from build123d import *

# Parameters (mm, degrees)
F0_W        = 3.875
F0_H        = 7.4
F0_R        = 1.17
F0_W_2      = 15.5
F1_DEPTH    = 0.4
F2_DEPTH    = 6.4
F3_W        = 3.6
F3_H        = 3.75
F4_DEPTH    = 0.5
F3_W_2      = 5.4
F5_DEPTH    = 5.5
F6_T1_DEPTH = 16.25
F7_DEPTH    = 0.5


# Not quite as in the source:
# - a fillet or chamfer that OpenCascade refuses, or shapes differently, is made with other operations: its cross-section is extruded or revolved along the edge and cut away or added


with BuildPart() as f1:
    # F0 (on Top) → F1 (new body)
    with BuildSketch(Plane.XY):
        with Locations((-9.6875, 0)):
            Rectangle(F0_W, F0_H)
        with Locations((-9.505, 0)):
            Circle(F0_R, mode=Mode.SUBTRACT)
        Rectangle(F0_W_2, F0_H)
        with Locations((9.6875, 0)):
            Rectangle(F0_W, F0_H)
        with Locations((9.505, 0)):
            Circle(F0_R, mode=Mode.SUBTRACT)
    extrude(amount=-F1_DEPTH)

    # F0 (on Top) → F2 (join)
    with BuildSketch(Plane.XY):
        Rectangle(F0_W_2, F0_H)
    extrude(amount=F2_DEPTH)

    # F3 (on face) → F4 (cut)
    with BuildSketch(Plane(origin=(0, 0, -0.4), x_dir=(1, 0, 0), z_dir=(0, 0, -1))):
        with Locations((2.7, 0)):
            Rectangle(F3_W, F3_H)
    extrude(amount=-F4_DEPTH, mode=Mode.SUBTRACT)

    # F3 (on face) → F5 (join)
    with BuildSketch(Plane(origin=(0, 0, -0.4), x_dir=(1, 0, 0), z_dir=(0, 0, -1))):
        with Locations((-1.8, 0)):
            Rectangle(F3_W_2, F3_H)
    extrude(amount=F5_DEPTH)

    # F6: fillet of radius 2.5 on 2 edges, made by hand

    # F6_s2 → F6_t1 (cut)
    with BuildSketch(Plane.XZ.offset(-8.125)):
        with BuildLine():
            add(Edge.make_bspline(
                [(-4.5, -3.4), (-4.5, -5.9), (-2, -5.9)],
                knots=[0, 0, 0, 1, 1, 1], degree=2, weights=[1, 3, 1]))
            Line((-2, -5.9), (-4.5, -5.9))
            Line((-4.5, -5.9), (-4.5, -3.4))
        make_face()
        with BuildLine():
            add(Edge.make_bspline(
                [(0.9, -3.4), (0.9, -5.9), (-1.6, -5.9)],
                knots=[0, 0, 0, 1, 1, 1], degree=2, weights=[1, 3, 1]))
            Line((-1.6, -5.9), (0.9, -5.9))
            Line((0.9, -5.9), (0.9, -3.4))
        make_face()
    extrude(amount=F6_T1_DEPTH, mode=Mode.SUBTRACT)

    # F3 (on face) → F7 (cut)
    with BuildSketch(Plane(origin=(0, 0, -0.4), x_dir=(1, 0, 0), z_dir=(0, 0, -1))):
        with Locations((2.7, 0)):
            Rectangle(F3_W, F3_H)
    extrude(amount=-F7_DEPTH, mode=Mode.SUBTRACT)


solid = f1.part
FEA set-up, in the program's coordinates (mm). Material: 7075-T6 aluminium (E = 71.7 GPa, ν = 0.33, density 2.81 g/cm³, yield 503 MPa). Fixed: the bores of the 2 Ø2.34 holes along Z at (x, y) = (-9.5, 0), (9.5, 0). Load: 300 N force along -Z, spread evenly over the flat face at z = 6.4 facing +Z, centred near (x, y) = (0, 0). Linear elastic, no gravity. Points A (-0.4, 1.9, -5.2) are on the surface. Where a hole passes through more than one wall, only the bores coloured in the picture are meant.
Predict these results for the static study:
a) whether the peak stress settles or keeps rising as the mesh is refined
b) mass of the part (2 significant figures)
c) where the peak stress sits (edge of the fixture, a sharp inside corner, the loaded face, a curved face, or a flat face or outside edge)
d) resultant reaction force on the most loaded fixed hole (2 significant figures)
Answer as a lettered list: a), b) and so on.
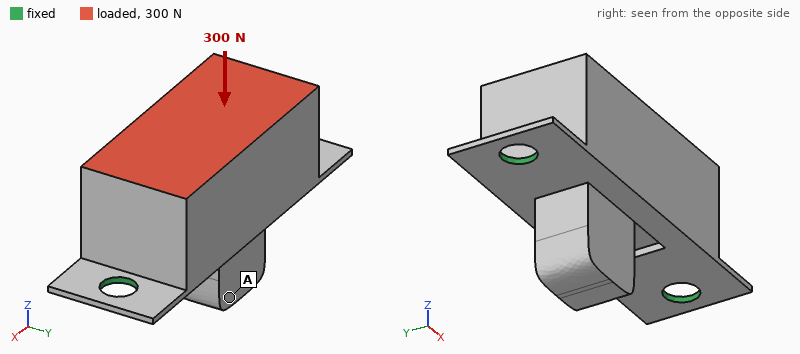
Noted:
a) keeps rising
b) 2.5 g
c) edge of the fixture
d) 180 N
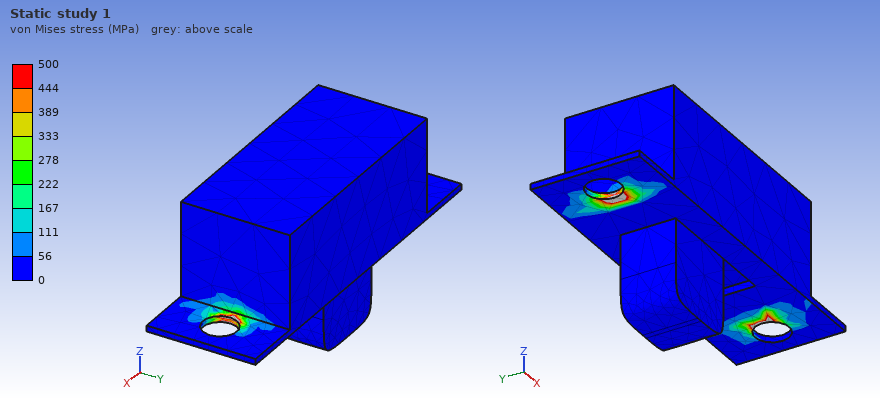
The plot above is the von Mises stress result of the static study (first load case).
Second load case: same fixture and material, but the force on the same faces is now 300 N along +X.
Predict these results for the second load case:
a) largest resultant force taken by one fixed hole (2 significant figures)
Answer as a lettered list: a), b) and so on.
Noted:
a) 190 N
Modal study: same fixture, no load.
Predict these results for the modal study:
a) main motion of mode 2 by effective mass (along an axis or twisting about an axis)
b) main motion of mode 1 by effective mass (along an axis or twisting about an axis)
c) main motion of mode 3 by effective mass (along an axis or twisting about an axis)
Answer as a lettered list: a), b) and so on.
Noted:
a) along Z
b) along Y
c) along X
